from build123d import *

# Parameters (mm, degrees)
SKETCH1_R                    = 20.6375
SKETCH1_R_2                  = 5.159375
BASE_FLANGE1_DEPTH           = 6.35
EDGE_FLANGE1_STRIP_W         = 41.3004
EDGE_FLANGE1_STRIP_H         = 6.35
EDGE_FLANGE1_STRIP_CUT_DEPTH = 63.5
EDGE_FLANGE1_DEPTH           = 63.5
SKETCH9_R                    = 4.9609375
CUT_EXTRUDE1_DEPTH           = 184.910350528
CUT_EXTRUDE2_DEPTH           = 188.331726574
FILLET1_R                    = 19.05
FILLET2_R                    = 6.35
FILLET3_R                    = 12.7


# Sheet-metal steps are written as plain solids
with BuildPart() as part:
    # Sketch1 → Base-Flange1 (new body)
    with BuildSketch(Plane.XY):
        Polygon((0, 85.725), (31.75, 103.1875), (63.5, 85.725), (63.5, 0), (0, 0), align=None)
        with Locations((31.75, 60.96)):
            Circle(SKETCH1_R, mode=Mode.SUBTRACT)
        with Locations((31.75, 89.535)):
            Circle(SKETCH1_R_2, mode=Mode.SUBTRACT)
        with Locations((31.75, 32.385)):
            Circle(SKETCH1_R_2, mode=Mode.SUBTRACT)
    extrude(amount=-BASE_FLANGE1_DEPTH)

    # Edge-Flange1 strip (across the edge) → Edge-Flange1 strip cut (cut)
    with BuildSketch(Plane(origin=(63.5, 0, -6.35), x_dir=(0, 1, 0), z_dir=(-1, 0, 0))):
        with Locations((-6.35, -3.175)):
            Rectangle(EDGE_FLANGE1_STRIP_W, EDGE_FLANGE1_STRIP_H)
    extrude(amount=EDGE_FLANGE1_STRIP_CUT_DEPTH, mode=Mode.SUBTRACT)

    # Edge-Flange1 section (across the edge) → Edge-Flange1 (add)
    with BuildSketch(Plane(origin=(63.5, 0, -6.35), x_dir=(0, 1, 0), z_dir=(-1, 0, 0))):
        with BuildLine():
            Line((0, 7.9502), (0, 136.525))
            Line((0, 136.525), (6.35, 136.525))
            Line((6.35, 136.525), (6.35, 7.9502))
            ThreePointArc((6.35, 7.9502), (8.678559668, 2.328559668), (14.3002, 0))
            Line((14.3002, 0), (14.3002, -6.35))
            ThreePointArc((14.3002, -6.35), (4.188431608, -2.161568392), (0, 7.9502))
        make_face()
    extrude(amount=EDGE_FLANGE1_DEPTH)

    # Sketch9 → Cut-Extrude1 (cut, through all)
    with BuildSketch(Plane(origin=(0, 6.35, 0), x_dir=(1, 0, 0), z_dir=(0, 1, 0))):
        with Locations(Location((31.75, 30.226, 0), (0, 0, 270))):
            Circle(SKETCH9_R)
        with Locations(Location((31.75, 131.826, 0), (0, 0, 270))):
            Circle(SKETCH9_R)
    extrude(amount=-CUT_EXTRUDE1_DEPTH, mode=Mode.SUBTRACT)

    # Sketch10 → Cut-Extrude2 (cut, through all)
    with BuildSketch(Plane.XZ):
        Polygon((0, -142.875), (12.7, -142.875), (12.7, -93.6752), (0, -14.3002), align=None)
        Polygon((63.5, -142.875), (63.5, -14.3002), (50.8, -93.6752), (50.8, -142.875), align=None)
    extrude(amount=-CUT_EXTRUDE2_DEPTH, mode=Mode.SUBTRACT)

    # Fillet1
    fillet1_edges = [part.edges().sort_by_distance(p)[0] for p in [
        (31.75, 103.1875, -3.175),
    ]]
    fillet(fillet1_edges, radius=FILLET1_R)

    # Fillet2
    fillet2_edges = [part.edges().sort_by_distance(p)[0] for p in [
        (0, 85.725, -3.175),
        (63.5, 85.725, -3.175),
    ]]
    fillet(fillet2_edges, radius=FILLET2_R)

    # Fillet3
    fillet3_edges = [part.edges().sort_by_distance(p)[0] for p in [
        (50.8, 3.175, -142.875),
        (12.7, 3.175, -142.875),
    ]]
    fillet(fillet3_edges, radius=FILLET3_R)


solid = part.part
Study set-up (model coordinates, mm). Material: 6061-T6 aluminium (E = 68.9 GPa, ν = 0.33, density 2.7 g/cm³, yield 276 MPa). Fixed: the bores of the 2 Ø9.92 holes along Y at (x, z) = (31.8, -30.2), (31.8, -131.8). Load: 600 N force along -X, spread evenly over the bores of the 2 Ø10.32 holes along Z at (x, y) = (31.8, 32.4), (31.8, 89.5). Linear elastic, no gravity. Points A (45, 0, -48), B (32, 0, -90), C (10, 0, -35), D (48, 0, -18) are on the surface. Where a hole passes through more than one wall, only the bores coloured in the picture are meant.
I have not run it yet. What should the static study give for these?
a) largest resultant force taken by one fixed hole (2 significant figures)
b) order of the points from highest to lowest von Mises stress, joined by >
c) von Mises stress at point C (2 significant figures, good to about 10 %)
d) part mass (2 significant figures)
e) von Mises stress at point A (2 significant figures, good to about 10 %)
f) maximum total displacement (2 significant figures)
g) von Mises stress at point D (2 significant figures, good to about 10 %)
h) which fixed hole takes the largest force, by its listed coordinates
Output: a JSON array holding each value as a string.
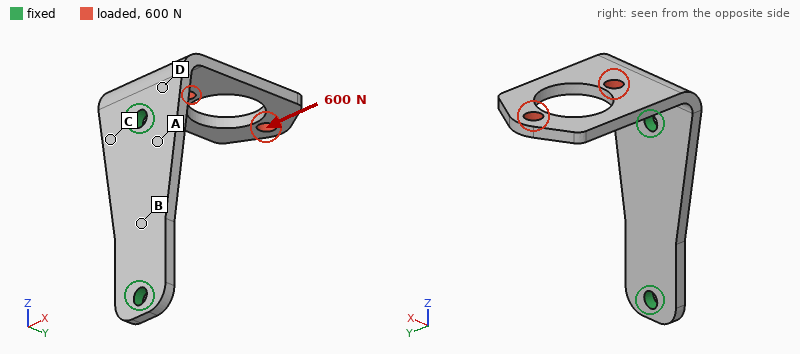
["720 N", "C > D > A > B", "40 MPa", "180 g", "18 MPa", "0.56 mm", "28 MPa", "(31.8, -30.2)"]
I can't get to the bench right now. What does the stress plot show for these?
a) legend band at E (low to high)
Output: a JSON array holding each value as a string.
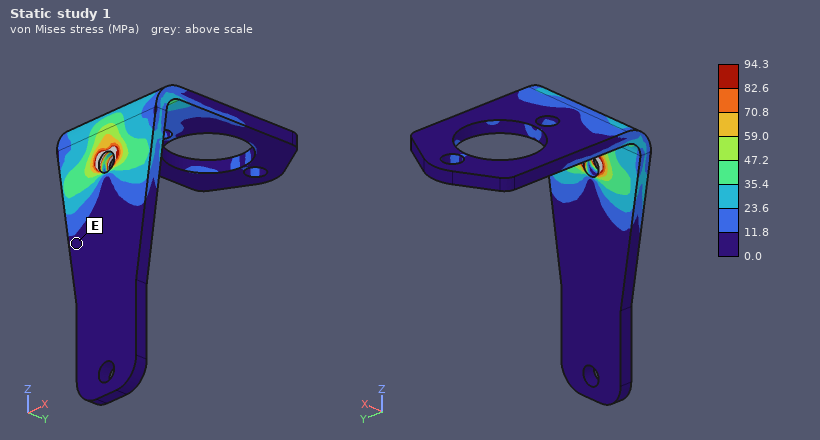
["0.0 to 11.8 MPa"]
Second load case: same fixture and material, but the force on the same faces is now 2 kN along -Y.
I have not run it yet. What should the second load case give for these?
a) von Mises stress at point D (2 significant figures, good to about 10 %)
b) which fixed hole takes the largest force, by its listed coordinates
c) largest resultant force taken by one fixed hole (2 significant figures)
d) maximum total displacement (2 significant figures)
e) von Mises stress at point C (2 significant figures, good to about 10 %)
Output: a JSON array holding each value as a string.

["57 MPa", "(31.8, -30.2)", "2.1 kN", "0.83 mm", "36 MPa"]
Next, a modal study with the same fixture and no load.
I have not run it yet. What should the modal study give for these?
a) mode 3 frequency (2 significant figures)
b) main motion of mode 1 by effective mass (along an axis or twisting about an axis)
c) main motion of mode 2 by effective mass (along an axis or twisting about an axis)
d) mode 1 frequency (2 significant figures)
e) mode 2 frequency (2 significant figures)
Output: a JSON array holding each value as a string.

["1700 Hz", "along Z", "along X", "500 Hz", "840 Hz"]
